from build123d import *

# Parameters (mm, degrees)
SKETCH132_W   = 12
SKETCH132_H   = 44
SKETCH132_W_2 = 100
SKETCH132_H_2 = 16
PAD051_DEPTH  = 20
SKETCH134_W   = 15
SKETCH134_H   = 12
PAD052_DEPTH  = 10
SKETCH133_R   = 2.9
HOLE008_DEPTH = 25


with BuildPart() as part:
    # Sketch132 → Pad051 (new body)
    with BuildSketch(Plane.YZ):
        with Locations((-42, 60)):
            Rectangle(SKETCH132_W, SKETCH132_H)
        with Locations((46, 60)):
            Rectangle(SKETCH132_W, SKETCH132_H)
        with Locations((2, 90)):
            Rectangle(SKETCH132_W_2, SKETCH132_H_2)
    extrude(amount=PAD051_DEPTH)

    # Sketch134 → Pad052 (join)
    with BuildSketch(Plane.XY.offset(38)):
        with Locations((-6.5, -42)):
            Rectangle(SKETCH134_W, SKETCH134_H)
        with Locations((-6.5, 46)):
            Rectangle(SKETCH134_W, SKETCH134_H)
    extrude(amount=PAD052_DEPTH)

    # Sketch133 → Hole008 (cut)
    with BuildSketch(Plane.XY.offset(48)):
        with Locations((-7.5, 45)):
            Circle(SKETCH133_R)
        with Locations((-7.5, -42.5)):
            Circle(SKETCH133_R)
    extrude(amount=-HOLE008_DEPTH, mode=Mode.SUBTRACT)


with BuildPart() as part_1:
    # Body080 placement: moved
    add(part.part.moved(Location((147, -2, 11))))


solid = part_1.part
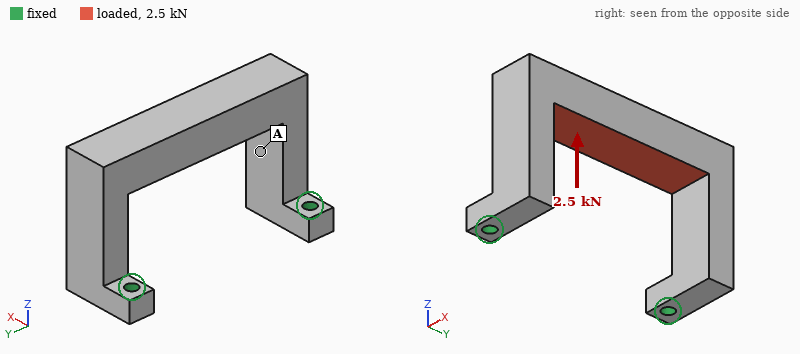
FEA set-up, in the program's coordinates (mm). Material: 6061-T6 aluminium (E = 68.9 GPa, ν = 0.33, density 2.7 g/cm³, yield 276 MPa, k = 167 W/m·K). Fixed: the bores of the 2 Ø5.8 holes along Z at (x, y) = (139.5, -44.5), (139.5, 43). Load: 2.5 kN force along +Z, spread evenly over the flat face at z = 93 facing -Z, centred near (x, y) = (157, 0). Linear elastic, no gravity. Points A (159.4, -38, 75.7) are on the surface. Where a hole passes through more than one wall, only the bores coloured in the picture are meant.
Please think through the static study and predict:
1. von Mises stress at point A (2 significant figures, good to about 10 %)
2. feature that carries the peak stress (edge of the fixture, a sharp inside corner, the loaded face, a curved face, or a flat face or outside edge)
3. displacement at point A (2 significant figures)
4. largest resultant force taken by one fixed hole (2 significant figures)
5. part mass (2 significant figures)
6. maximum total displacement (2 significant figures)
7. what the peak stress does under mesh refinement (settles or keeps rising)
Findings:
15 MPa
edge of the fixture
0.063 mm
1.3 kN
150 g
0.15 mm
keeps rising
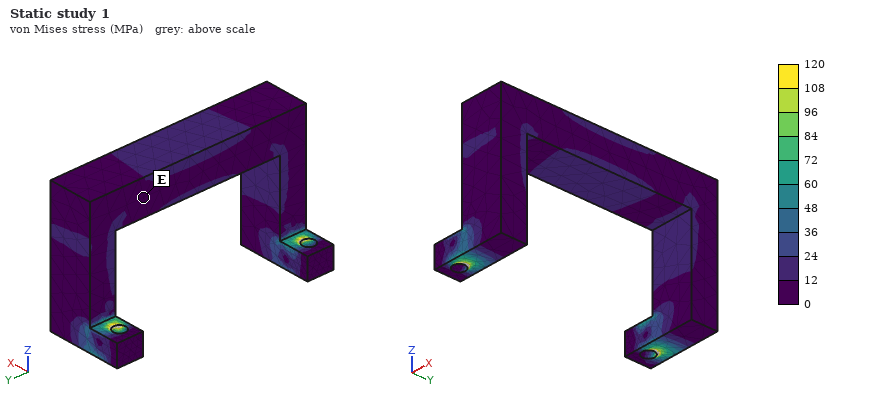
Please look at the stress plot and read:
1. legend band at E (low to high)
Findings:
0 to 12 MPa
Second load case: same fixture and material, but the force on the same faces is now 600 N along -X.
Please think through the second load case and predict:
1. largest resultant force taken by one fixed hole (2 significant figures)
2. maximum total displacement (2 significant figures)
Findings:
300 N
0.13 mm
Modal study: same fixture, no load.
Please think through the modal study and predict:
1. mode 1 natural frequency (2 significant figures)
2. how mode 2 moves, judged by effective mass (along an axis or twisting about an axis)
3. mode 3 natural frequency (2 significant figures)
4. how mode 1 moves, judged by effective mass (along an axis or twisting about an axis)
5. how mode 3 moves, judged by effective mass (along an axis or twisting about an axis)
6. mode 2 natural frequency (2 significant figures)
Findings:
1100 Hz
along Y
2600 Hz
along X
twisting about Z
1900 Hz
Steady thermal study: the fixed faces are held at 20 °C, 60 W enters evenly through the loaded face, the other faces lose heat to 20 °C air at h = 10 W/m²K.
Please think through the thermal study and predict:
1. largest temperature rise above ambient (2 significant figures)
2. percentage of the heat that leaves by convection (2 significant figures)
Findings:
57 K
7.3 %
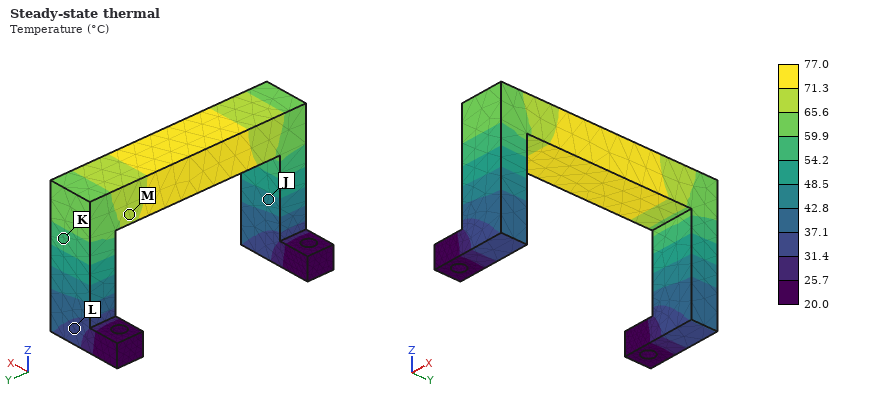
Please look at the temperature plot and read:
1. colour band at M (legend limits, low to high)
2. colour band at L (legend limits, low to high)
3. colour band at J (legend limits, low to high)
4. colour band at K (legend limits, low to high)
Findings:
65.6 to 71.3 °C
31.4 to 37.1 °C
42.8 to 48.5 °C
54.2 to 59.9 °C
